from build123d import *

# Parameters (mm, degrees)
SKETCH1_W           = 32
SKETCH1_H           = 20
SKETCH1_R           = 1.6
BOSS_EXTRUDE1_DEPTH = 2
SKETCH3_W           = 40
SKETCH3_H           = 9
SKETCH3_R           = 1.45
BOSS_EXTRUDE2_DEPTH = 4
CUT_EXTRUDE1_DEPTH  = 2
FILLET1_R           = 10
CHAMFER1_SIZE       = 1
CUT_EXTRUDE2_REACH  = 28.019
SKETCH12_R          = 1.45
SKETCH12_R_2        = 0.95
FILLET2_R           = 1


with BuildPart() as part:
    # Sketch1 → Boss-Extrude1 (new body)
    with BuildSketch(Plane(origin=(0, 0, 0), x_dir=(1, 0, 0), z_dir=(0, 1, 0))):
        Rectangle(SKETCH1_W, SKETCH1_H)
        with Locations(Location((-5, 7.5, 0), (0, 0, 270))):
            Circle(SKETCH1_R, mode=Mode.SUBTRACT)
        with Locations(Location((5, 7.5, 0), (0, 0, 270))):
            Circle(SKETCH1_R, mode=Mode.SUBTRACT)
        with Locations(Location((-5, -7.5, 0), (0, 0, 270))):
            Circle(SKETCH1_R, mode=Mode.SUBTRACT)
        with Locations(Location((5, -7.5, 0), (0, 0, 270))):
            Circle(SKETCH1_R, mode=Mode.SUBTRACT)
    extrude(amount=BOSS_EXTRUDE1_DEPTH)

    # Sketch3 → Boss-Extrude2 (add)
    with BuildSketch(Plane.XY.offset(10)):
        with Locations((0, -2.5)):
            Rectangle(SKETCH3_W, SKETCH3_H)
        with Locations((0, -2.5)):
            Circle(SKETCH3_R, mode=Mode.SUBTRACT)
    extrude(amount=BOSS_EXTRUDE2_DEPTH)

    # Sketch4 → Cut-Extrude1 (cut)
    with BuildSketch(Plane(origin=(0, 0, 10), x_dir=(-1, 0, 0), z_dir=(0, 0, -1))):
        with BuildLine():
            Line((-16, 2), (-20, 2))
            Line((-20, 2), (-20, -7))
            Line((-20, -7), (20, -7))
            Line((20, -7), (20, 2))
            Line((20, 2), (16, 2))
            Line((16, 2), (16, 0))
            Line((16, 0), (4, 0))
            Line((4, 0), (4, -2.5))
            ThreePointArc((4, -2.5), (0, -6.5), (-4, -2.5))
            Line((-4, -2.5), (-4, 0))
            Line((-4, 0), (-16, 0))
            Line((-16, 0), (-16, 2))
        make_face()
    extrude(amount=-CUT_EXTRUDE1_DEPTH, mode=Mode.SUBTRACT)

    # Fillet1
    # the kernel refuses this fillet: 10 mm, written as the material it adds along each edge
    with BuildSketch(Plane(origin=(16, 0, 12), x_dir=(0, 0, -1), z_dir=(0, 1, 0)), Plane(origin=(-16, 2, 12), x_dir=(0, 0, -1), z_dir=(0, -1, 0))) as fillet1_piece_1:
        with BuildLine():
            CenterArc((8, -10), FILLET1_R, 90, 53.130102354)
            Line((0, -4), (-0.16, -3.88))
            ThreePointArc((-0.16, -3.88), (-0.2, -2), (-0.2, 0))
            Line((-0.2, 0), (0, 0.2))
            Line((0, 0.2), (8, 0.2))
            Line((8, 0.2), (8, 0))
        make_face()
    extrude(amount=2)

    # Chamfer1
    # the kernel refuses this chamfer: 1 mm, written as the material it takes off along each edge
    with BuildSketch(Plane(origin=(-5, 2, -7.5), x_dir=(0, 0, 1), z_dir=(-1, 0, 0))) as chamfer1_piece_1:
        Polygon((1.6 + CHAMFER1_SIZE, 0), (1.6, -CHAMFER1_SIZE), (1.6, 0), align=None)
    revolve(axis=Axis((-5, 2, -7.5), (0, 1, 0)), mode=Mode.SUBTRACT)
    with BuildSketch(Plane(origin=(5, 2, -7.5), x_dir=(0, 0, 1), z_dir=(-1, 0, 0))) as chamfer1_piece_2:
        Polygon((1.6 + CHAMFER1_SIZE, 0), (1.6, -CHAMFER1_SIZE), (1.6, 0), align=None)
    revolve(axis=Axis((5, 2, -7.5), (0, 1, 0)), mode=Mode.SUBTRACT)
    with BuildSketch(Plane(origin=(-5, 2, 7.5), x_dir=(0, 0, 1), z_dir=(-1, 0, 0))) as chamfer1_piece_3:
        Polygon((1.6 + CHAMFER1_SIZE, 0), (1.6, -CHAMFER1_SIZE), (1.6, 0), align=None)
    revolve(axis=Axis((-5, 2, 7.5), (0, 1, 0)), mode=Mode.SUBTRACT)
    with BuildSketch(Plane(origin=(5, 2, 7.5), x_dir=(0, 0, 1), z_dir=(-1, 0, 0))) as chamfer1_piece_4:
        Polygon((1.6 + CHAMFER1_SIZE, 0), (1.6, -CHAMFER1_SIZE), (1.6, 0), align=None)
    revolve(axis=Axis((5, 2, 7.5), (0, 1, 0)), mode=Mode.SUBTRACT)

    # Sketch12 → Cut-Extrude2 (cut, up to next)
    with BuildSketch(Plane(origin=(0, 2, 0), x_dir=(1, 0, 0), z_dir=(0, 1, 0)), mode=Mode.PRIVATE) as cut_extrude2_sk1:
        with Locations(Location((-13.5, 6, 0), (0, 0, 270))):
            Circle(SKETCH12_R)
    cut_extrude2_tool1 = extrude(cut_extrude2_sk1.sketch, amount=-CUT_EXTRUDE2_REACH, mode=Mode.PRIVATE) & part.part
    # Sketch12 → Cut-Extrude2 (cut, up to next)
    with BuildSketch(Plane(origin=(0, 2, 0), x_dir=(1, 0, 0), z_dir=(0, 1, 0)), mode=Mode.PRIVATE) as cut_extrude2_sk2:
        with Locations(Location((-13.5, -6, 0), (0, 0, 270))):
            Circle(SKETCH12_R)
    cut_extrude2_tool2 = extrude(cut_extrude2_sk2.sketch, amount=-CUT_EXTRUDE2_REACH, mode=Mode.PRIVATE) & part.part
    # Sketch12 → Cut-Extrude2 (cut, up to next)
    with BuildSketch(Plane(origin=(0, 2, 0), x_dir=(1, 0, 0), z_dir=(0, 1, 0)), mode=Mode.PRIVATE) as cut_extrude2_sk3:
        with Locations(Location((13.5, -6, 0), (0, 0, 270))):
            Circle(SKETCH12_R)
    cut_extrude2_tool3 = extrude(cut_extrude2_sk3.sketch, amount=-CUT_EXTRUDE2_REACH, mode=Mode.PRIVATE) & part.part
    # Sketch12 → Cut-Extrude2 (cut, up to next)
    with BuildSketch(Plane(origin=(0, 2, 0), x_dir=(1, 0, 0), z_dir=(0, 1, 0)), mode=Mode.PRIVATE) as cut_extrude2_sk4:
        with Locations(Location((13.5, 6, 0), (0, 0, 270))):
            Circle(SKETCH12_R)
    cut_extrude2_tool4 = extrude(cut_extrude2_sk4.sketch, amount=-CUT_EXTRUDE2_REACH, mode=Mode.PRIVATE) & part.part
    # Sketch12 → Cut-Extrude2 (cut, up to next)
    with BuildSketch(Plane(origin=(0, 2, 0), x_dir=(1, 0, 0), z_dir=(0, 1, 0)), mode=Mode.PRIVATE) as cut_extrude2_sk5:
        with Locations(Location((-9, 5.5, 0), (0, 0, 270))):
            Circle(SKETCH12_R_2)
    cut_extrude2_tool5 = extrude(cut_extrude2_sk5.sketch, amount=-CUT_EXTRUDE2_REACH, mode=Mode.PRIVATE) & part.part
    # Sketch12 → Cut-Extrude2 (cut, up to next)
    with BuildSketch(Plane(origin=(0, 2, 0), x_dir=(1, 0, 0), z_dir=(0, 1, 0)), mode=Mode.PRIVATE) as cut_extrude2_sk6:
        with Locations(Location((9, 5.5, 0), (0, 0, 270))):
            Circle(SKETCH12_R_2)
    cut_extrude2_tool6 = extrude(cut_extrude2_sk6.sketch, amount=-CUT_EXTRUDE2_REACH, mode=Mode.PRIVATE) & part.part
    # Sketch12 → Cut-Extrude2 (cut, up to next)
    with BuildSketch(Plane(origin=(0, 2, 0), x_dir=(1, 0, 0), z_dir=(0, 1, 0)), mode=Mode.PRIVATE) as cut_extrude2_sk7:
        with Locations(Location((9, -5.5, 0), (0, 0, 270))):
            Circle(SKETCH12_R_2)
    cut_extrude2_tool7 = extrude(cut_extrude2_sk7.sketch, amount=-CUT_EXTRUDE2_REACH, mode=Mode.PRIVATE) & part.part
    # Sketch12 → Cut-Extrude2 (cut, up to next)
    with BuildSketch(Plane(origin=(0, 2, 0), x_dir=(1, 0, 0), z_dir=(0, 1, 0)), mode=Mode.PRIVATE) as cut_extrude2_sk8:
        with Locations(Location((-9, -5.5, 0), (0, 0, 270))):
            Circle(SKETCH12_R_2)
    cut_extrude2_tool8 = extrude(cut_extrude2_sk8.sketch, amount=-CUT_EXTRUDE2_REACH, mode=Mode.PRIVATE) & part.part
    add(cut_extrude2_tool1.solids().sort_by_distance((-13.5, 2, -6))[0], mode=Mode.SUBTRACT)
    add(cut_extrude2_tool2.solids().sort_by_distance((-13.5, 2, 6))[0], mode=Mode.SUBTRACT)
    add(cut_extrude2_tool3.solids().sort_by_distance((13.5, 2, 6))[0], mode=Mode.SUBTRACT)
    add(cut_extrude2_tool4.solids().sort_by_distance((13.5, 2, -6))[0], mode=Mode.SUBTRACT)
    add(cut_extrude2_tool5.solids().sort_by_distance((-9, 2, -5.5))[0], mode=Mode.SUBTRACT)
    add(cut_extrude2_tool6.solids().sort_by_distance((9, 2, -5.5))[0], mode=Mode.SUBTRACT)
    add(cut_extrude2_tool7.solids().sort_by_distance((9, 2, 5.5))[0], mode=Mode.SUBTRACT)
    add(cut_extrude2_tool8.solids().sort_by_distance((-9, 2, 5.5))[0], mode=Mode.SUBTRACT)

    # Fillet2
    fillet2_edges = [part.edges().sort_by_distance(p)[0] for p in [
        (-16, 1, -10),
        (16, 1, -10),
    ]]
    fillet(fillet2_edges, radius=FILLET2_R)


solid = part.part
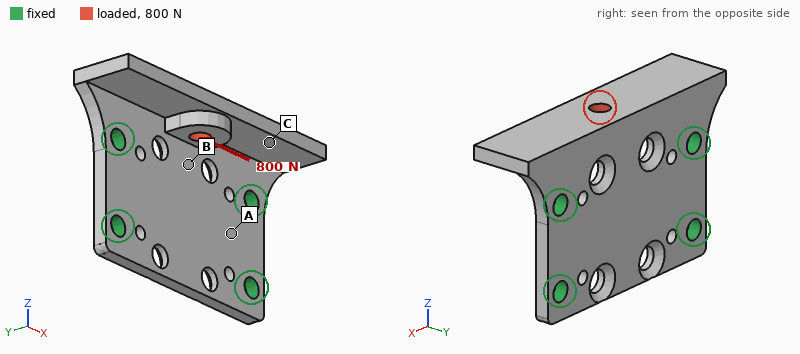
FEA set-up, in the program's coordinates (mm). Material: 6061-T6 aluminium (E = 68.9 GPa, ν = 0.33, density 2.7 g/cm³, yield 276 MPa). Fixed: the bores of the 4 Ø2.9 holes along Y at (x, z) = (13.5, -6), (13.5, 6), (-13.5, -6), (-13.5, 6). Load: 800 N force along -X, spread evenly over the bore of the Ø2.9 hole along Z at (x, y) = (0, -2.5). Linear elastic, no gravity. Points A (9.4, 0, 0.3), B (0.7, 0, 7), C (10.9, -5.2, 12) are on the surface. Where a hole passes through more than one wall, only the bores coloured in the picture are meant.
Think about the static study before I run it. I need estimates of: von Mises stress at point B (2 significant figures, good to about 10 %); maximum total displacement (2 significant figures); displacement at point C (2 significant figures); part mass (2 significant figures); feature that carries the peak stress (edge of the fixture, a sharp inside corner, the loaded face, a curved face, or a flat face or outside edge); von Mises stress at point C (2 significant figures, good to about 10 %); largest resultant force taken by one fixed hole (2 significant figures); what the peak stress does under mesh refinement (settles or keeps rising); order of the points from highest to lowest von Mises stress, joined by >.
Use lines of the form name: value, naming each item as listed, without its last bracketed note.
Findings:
von Mises stress at point B: 42 MPa
maximum total displacement: 29 µm
displacement at point C: 18 µm
part mass: 5.6 g
feature that carries the peak stress: edge of the fixture
von Mises stress at point C: 19 MPa
largest resultant force taken by one fixed hole: 390 N
what the peak stress does under mesh refinement: keeps rising
order of the points from highest to lowest von Mises stress, joined by >: B > C > A
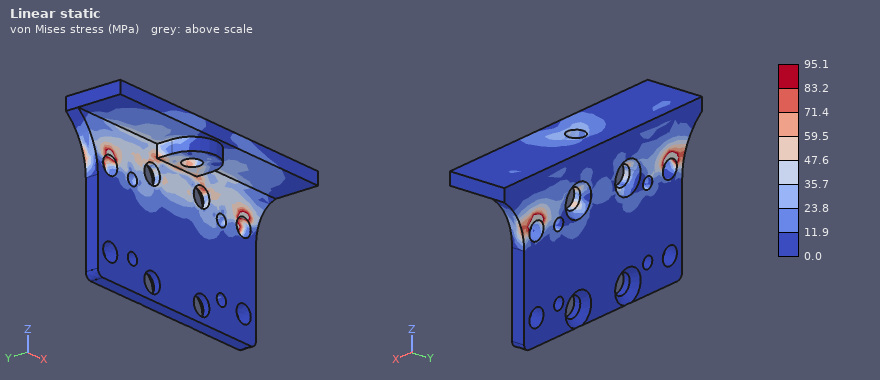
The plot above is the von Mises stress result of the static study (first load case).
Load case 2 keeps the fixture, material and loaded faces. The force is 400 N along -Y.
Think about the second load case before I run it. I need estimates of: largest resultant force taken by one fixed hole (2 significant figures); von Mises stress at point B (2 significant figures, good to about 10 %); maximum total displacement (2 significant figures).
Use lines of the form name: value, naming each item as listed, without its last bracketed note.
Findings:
largest resultant force taken by one fixed hole: 240 N
von Mises stress at point B: 35 MPa
maximum total displacement: 61 µm
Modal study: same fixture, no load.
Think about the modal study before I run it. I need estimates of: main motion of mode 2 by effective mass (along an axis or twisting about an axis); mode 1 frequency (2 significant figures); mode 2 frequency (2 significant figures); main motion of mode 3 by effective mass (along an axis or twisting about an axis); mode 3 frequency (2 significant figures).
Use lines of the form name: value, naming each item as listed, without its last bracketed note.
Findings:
main motion of mode 2 by effective mass: twisting about Z
mode 1 frequency: 8300 Hz
mode 2 frequency: 12 kHz
main motion of mode 3 by effective mass: along Y
mode 3 frequency: 16 kHz
